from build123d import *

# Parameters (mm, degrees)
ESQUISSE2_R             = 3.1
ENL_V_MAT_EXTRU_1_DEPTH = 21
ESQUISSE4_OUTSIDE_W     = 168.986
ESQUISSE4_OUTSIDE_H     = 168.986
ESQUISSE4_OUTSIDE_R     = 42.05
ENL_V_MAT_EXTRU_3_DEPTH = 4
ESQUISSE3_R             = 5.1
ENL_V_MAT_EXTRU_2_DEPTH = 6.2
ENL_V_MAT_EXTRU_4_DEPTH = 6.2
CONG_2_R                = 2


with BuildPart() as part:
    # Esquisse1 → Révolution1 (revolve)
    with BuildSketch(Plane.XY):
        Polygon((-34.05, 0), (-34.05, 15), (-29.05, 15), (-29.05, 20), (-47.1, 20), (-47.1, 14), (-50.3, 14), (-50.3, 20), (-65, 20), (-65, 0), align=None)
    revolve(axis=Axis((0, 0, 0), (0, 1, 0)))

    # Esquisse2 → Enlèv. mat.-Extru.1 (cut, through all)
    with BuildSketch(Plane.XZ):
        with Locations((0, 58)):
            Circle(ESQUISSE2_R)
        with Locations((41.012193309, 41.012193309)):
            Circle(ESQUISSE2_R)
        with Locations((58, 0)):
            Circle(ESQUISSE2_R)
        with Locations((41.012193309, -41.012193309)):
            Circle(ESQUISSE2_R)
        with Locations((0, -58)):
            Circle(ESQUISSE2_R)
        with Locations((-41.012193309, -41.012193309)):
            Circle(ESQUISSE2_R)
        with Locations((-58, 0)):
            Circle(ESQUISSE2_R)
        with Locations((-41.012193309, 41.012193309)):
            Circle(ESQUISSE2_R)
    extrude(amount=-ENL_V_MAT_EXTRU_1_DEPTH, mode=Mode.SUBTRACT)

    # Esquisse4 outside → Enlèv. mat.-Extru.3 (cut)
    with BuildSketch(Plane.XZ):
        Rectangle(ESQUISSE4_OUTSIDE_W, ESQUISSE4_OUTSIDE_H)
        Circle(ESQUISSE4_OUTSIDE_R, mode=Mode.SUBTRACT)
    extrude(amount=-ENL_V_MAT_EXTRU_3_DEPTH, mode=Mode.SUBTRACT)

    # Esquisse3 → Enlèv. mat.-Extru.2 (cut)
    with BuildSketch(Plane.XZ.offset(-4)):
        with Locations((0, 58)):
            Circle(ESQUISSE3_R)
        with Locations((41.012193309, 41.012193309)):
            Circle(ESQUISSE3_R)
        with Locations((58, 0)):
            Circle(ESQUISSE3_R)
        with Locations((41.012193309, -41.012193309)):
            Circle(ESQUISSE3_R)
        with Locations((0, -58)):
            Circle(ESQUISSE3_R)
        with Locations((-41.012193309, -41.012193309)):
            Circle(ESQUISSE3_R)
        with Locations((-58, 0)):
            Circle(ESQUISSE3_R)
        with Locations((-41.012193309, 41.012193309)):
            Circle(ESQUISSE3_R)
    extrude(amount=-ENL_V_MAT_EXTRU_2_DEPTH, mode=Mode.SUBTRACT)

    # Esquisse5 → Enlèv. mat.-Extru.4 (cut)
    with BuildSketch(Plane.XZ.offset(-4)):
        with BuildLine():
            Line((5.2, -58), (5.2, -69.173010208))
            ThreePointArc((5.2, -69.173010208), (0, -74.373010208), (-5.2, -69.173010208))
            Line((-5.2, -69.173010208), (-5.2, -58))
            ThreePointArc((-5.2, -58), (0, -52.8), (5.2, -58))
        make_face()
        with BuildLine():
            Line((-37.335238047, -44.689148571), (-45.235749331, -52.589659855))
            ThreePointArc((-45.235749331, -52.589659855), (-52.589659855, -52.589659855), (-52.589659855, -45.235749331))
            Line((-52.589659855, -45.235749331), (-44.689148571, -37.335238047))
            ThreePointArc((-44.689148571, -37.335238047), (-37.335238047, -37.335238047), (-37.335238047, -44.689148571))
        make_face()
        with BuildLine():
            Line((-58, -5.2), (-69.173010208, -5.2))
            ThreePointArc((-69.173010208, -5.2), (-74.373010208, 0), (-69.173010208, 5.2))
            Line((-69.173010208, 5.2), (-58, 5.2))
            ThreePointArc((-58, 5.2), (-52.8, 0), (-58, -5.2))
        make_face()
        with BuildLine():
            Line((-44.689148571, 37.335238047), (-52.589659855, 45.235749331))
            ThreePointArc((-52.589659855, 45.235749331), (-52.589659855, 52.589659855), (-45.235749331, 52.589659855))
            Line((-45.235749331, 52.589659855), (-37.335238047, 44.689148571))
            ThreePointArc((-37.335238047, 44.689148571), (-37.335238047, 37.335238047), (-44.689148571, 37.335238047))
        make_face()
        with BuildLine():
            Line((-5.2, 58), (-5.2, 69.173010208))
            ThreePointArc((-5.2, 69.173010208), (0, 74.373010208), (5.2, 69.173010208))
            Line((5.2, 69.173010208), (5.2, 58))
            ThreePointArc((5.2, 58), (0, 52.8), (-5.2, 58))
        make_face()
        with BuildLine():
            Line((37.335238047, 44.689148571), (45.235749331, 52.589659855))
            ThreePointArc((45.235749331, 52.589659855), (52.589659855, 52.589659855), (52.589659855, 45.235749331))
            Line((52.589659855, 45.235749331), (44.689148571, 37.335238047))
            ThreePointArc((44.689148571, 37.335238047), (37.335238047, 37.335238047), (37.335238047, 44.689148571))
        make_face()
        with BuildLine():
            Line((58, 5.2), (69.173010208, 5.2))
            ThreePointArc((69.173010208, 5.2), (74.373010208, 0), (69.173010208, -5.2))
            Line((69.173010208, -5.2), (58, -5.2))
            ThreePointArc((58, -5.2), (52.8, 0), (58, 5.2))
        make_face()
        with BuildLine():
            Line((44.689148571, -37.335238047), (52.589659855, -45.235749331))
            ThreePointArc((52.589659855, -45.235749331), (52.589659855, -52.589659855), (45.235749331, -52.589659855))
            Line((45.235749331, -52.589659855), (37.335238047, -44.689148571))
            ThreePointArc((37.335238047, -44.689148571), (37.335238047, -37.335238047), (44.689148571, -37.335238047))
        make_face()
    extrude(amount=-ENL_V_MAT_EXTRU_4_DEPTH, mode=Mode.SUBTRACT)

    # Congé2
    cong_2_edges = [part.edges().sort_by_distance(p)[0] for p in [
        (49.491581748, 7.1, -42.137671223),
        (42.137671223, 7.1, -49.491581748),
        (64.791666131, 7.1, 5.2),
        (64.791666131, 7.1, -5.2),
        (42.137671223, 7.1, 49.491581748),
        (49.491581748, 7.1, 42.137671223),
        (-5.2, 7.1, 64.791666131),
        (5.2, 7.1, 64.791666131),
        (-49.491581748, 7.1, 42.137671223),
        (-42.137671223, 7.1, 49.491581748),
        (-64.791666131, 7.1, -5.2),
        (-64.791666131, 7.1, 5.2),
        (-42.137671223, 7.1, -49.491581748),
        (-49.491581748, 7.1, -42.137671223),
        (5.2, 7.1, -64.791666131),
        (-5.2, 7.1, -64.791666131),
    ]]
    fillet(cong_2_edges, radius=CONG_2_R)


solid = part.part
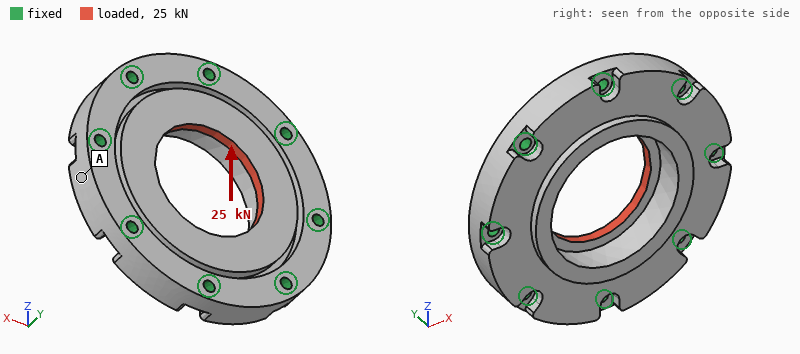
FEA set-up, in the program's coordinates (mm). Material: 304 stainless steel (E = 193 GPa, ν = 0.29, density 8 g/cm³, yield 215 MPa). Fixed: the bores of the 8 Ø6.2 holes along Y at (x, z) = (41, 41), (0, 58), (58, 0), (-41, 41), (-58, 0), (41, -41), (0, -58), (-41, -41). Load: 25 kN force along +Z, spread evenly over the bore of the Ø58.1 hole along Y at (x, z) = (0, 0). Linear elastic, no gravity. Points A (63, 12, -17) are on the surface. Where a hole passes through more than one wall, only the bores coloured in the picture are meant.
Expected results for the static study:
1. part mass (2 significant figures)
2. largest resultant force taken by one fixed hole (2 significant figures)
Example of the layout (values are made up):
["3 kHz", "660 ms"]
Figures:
["1.2 kg", "4.0 kN"]
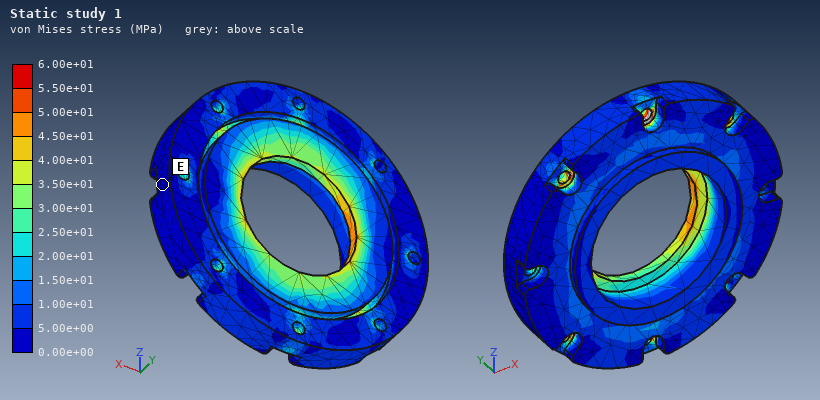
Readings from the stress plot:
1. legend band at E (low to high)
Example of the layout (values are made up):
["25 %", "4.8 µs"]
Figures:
["0.00e+00 to 5.00e+00 MPa"]
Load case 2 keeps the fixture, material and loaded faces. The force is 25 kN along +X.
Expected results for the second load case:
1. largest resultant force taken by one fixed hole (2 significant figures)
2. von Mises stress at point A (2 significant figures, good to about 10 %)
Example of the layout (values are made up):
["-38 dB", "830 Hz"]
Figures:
["4.0 kN", "8.3 MPa"]
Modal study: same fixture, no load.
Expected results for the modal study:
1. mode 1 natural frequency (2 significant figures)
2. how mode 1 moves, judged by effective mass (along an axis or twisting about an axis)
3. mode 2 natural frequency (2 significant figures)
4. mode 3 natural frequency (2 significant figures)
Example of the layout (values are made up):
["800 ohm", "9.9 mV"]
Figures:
["9300 Hz", "along Y", "12 kHz", "12 kHz"]
